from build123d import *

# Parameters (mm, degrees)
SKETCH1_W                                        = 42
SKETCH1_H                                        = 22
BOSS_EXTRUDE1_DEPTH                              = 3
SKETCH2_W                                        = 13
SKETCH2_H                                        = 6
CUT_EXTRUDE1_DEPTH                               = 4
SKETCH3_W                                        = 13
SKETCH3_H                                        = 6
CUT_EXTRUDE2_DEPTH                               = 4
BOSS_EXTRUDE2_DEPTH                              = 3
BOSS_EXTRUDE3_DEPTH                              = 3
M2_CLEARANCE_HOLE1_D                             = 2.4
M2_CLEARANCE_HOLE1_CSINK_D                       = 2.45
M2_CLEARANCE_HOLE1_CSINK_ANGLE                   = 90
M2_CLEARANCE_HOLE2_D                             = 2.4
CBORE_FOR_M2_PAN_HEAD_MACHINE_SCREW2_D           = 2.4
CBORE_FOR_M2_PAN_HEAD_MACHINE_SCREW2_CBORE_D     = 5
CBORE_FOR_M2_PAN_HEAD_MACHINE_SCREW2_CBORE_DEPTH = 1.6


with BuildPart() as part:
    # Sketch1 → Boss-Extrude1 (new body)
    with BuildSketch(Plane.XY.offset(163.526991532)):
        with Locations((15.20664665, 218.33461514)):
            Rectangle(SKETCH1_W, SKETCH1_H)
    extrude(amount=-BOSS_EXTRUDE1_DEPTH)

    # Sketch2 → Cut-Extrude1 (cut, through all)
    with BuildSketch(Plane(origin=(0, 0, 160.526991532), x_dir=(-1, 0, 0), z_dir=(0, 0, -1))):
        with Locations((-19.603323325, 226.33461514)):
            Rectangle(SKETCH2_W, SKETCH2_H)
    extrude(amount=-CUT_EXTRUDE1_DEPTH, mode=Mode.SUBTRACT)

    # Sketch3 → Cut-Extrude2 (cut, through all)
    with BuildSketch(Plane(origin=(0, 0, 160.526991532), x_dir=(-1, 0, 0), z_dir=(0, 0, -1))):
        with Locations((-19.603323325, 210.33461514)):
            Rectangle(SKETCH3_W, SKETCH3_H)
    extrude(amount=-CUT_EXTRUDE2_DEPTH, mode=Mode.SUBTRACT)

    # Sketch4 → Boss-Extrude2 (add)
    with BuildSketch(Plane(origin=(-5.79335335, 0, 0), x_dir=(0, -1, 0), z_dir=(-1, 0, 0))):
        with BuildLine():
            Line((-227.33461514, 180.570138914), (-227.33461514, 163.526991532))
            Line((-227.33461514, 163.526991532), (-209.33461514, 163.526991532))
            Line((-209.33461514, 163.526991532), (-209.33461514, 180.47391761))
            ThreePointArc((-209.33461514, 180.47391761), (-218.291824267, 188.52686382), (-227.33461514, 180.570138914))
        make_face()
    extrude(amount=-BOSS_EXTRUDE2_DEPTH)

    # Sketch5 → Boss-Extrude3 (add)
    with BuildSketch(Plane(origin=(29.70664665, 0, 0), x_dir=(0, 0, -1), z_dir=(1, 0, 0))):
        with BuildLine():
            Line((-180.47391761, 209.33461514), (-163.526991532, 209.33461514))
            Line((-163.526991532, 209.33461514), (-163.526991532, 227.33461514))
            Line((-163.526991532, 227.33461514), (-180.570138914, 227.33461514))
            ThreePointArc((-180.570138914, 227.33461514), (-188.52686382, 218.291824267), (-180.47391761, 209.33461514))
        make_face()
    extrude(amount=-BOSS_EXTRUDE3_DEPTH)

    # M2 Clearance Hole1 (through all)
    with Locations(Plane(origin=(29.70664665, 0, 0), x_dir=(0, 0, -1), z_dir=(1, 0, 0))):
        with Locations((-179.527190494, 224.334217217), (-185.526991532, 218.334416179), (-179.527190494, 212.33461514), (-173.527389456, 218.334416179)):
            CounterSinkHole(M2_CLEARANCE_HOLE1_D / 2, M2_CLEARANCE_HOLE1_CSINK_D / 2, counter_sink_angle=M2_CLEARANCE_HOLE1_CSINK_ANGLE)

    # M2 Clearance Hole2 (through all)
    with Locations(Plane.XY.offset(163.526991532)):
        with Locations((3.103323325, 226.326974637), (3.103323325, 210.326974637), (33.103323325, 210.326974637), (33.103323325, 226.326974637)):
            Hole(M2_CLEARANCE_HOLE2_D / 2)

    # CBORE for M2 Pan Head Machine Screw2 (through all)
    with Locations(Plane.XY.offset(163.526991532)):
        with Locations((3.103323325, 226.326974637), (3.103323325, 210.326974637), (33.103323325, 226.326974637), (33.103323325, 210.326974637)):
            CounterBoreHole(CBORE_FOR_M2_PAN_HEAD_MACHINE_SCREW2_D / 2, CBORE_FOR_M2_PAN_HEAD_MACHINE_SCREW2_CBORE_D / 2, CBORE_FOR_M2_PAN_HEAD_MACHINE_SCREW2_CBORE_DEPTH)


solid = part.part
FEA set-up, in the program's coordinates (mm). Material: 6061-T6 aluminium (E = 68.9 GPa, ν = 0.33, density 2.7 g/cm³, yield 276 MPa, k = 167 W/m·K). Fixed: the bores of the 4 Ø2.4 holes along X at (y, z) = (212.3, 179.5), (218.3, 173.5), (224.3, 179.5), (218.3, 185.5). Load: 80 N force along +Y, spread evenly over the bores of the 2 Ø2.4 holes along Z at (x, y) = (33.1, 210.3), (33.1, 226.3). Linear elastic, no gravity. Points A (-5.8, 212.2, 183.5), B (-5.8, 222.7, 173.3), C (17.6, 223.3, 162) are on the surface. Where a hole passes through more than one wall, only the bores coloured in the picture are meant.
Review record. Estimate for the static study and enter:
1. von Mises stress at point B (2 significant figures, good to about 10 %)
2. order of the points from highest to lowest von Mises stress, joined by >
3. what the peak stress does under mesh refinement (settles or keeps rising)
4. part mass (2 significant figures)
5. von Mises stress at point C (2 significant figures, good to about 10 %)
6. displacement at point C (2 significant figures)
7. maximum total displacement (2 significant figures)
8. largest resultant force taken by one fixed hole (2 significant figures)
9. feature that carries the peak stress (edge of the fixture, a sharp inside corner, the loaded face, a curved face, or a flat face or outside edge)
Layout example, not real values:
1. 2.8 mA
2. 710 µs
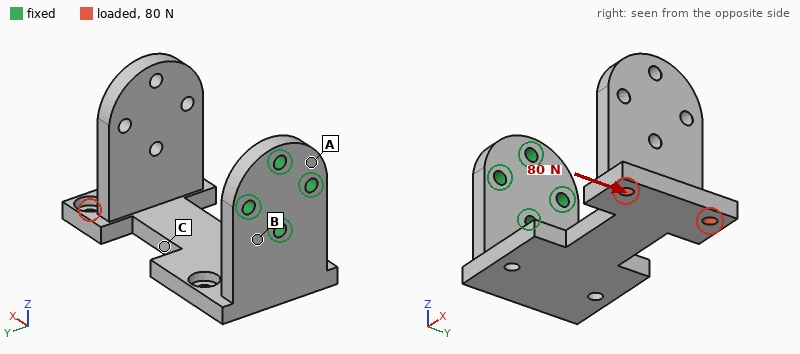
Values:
1. 64 MPa
2. B > C > A
3. keeps rising
4. 12 g
5. 25 MPa
6. 0.17 mm
7. 0.33 mm
8. 110 N
9. edge of the fixture
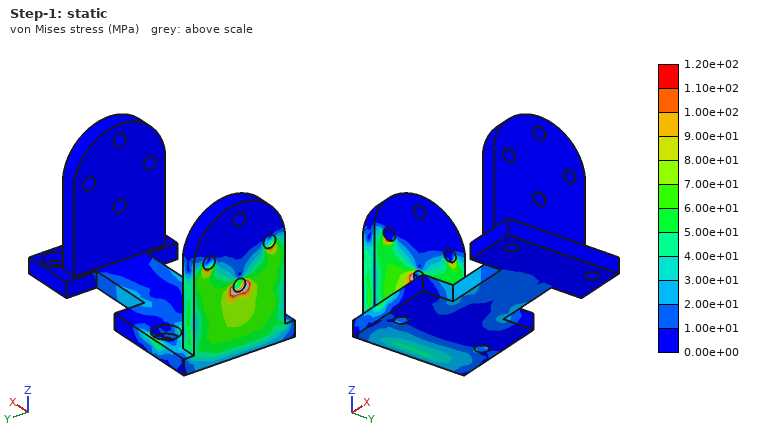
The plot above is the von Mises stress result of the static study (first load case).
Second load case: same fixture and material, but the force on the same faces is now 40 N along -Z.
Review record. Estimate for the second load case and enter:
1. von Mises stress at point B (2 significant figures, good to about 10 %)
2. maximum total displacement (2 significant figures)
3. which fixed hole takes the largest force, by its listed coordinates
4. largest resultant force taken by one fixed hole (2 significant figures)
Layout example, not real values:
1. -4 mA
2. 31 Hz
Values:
1. 31 MPa
2. 0.61 mm
3. (218.3, 173.5)
4. 130 N
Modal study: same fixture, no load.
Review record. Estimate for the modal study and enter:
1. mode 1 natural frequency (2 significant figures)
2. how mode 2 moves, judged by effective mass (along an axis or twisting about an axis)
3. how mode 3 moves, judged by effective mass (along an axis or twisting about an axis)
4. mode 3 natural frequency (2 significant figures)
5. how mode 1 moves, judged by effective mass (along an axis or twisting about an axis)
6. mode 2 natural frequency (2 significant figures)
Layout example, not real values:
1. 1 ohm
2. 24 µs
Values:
1. 660 Hz
2. along Y
3. along X
4. 2100 Hz
5. along Z
6. 1000 Hz
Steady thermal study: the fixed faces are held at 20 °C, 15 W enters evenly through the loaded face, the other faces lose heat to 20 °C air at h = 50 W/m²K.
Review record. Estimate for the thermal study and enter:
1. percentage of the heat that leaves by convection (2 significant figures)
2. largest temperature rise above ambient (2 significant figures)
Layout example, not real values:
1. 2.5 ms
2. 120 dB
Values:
1. 45 %
2. 75 K
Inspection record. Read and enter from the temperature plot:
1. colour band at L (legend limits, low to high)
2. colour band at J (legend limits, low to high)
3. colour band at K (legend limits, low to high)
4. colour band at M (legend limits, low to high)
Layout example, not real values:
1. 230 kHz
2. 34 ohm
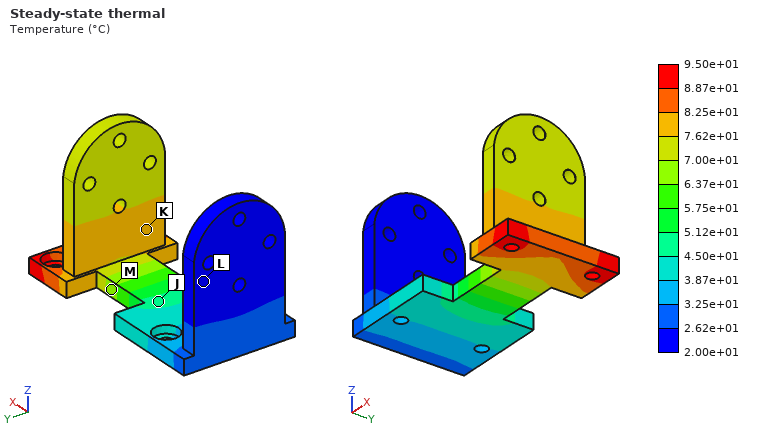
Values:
1. 2.00e+01 to 2.62e+01 °C
2. 4.50e+01 to 5.12e+01 °C
3. 7.62e+01 to 8.25e+01 °C
4. 6.37e+01 to 7.00e+01 °C
